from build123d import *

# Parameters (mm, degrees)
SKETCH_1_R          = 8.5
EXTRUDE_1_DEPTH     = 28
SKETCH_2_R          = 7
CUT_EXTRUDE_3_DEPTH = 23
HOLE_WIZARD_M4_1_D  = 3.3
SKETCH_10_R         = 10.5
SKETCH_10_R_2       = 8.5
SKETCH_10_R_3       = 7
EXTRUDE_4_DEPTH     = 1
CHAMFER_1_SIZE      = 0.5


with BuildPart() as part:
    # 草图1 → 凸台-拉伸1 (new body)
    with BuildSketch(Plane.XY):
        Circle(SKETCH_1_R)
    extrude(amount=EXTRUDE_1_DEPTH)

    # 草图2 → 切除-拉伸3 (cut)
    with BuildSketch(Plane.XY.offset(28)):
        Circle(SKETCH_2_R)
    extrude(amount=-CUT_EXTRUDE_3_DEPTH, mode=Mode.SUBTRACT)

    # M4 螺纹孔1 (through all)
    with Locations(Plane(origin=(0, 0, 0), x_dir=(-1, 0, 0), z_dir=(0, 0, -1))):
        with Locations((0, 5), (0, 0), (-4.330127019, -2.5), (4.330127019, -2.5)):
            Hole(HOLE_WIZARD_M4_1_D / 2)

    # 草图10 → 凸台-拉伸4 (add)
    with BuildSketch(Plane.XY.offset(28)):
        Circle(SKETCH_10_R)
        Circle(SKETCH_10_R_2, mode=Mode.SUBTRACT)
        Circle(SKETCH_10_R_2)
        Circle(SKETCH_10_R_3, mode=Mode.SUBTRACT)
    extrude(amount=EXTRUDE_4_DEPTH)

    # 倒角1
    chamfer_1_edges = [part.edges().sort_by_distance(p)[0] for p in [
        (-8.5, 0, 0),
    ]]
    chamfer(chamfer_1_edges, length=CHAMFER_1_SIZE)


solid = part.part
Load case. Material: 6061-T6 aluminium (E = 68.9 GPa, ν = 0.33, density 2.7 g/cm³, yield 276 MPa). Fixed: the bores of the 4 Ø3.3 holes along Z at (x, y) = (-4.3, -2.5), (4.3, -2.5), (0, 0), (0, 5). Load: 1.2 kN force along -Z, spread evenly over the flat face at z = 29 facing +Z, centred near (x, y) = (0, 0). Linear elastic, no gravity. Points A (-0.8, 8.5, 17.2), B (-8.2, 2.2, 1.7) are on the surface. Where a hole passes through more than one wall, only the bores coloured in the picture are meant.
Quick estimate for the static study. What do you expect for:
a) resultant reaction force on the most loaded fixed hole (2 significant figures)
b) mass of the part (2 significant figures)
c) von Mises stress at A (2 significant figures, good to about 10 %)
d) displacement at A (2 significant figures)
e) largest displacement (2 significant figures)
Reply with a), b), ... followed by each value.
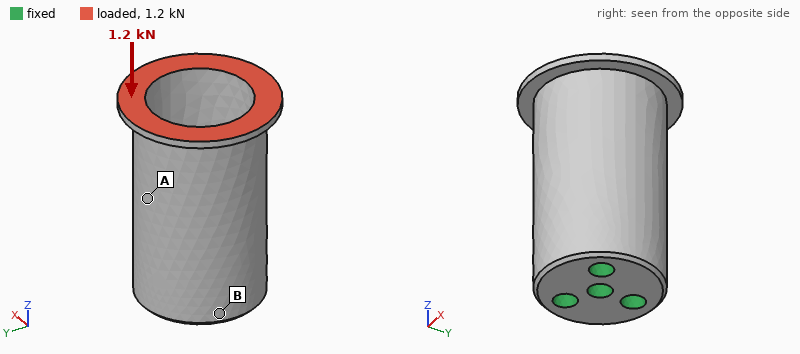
a) 390 N
b) 7.6 g
c) 16 MPa
d) 4.2 µm
e) 16 µm
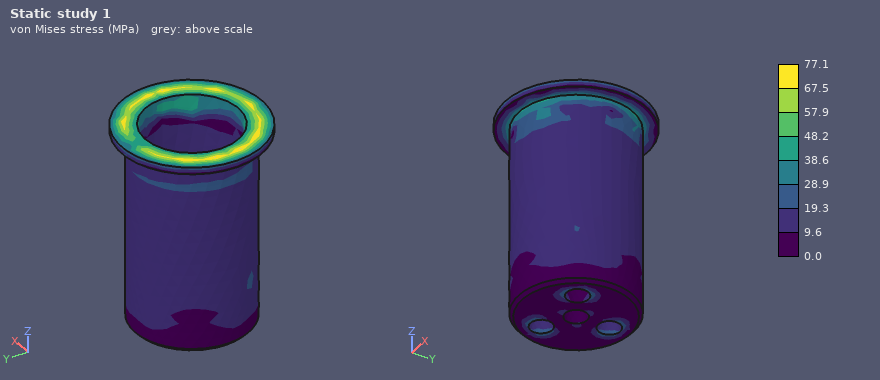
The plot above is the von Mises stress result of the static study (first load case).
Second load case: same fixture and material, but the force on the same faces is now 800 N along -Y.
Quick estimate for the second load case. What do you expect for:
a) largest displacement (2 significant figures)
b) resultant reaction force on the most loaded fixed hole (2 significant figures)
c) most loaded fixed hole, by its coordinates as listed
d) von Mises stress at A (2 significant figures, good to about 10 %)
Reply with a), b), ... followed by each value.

a) 74 µm
b) 1.5 kN
c) (0, 5)
d) 39 MPa
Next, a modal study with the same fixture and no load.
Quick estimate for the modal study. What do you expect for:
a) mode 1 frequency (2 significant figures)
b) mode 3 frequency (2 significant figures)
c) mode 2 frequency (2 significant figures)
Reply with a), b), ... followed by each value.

a) 13 kHz
b) 21 kHz
c) 13 kHz
